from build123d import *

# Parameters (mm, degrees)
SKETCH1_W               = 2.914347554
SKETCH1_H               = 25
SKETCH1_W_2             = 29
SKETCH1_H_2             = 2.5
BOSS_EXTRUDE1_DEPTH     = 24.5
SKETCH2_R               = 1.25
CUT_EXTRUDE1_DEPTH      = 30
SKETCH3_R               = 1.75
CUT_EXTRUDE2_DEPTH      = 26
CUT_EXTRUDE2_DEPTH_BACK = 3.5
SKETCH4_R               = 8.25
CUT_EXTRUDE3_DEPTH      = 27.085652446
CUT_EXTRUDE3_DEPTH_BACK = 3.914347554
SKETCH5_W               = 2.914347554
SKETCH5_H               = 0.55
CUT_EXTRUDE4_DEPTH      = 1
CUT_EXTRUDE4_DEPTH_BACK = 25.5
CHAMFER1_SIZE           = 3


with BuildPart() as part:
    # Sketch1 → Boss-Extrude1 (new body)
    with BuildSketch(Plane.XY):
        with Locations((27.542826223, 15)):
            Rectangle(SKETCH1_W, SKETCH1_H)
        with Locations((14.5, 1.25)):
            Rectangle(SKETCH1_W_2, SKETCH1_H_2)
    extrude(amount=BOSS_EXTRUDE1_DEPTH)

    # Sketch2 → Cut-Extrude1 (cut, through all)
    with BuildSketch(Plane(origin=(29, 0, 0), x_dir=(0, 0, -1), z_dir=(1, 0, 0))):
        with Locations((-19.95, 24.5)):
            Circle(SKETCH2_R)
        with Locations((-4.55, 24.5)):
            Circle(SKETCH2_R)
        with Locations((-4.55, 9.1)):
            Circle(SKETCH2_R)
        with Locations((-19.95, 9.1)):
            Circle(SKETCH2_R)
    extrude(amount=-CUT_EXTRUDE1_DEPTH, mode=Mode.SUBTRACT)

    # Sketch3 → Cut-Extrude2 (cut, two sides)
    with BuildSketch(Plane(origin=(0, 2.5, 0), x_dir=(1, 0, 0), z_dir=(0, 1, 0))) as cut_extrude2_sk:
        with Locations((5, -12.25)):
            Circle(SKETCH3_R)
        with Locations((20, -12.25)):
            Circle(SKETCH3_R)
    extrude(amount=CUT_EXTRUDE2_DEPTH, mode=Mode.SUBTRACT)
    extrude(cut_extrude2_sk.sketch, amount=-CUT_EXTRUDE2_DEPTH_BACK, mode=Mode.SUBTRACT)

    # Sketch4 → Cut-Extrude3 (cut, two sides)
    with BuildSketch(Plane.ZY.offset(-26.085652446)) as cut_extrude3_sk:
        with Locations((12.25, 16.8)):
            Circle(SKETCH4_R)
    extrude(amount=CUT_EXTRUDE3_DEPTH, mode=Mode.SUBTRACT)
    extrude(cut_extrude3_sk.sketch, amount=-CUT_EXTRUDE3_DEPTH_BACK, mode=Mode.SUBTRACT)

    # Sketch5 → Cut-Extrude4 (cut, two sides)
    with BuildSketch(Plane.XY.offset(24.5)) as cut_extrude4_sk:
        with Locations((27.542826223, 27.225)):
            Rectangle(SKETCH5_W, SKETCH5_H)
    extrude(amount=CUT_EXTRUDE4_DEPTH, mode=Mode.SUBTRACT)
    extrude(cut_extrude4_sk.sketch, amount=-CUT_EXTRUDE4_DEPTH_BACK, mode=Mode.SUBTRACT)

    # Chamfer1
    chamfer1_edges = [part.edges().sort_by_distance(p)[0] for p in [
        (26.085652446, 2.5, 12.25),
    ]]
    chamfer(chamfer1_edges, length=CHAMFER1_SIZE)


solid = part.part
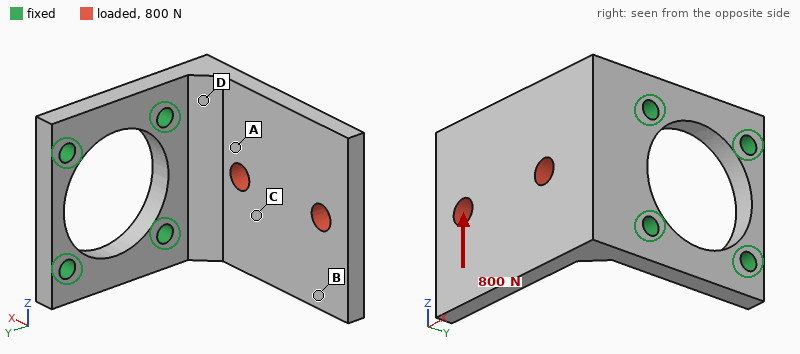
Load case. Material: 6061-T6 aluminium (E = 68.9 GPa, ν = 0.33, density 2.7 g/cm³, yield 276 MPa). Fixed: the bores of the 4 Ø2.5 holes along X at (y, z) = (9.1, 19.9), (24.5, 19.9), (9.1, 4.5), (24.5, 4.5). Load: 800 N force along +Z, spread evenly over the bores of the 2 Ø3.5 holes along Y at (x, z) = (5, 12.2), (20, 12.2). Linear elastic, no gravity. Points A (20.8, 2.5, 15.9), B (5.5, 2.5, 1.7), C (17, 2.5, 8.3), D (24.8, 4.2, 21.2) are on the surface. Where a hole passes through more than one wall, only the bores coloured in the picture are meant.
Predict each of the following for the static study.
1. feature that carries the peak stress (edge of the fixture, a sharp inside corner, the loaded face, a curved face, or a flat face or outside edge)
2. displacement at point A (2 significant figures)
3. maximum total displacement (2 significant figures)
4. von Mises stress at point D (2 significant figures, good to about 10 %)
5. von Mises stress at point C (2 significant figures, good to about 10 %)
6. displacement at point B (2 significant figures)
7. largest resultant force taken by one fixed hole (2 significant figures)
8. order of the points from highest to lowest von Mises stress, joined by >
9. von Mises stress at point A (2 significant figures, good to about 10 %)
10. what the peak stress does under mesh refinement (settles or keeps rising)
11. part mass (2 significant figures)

edge of the fixture
0.033 mm
0.14 mm
85 MPa
32 MPa
0.11 mm
860 N
D > A > C > B
63 MPa
keeps rising
7.8 g
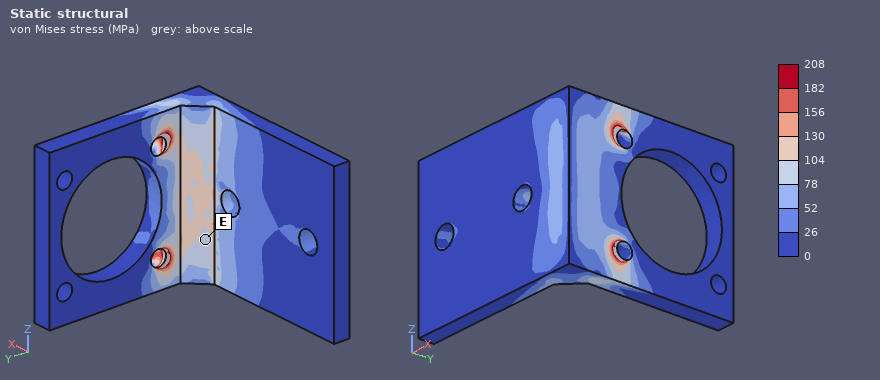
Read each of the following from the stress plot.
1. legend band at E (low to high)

78 to 104 MPa
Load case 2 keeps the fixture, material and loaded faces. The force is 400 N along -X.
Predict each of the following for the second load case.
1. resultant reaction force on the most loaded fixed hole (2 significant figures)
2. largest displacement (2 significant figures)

210 N
0.11 mm
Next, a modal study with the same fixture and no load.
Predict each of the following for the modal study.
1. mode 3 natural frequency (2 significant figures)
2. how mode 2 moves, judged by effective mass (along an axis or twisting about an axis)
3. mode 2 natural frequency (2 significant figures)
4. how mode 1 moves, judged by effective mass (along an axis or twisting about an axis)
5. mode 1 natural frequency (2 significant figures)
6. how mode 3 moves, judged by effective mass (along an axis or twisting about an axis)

8700 Hz
along Z
6300 Hz
along Y
2400 Hz
along Z
